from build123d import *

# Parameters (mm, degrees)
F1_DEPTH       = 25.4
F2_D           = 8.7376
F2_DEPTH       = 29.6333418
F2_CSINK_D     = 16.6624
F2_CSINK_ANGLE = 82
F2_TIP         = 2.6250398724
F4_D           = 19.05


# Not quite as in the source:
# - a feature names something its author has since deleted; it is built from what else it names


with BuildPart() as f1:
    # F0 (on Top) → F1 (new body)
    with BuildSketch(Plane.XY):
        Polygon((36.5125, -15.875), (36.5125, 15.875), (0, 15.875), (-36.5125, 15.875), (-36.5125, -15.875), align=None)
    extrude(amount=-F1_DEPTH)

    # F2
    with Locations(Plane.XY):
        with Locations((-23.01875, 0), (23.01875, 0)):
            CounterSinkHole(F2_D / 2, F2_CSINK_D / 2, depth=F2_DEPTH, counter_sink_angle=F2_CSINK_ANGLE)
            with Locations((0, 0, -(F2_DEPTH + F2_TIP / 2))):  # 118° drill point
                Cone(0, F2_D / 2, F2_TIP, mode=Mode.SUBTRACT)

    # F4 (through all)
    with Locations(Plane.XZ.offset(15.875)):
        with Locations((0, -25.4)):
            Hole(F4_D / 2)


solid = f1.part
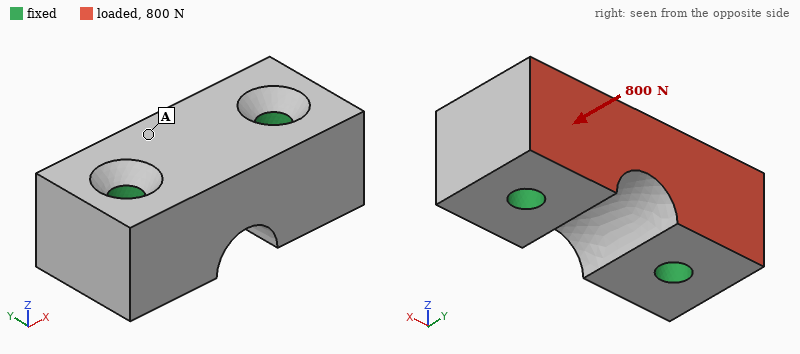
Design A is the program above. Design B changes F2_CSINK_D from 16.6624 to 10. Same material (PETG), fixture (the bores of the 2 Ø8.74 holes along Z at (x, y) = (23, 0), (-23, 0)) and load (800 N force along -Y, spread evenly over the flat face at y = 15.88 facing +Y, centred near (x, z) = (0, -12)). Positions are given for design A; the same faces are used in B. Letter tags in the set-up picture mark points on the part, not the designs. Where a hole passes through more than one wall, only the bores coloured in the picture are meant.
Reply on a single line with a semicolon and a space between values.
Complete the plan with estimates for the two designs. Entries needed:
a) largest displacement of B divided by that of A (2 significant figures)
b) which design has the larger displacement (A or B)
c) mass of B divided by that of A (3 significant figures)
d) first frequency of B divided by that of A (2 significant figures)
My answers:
0.78; A; 1.01; 1.1
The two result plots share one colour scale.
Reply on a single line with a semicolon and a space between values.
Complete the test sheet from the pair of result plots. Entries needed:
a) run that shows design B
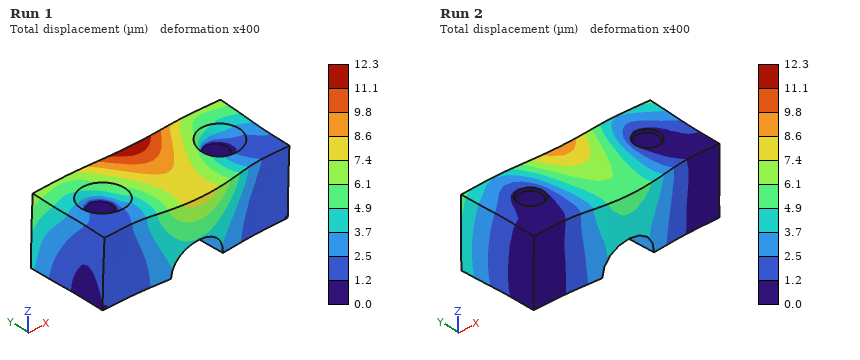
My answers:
Run 2
